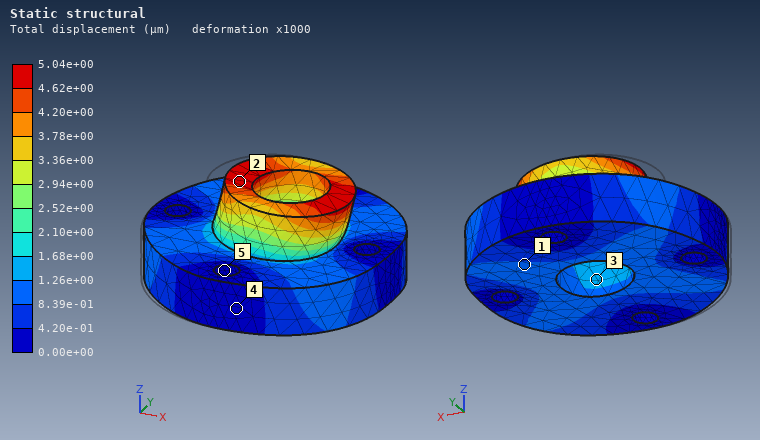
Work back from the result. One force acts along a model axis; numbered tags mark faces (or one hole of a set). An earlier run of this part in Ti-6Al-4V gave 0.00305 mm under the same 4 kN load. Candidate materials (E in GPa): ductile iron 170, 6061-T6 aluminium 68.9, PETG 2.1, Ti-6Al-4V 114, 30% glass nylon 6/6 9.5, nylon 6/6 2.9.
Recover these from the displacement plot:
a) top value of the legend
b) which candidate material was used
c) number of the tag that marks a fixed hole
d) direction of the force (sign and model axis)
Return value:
5.04e+00 µm
6061-T6 aluminium
5
+X
